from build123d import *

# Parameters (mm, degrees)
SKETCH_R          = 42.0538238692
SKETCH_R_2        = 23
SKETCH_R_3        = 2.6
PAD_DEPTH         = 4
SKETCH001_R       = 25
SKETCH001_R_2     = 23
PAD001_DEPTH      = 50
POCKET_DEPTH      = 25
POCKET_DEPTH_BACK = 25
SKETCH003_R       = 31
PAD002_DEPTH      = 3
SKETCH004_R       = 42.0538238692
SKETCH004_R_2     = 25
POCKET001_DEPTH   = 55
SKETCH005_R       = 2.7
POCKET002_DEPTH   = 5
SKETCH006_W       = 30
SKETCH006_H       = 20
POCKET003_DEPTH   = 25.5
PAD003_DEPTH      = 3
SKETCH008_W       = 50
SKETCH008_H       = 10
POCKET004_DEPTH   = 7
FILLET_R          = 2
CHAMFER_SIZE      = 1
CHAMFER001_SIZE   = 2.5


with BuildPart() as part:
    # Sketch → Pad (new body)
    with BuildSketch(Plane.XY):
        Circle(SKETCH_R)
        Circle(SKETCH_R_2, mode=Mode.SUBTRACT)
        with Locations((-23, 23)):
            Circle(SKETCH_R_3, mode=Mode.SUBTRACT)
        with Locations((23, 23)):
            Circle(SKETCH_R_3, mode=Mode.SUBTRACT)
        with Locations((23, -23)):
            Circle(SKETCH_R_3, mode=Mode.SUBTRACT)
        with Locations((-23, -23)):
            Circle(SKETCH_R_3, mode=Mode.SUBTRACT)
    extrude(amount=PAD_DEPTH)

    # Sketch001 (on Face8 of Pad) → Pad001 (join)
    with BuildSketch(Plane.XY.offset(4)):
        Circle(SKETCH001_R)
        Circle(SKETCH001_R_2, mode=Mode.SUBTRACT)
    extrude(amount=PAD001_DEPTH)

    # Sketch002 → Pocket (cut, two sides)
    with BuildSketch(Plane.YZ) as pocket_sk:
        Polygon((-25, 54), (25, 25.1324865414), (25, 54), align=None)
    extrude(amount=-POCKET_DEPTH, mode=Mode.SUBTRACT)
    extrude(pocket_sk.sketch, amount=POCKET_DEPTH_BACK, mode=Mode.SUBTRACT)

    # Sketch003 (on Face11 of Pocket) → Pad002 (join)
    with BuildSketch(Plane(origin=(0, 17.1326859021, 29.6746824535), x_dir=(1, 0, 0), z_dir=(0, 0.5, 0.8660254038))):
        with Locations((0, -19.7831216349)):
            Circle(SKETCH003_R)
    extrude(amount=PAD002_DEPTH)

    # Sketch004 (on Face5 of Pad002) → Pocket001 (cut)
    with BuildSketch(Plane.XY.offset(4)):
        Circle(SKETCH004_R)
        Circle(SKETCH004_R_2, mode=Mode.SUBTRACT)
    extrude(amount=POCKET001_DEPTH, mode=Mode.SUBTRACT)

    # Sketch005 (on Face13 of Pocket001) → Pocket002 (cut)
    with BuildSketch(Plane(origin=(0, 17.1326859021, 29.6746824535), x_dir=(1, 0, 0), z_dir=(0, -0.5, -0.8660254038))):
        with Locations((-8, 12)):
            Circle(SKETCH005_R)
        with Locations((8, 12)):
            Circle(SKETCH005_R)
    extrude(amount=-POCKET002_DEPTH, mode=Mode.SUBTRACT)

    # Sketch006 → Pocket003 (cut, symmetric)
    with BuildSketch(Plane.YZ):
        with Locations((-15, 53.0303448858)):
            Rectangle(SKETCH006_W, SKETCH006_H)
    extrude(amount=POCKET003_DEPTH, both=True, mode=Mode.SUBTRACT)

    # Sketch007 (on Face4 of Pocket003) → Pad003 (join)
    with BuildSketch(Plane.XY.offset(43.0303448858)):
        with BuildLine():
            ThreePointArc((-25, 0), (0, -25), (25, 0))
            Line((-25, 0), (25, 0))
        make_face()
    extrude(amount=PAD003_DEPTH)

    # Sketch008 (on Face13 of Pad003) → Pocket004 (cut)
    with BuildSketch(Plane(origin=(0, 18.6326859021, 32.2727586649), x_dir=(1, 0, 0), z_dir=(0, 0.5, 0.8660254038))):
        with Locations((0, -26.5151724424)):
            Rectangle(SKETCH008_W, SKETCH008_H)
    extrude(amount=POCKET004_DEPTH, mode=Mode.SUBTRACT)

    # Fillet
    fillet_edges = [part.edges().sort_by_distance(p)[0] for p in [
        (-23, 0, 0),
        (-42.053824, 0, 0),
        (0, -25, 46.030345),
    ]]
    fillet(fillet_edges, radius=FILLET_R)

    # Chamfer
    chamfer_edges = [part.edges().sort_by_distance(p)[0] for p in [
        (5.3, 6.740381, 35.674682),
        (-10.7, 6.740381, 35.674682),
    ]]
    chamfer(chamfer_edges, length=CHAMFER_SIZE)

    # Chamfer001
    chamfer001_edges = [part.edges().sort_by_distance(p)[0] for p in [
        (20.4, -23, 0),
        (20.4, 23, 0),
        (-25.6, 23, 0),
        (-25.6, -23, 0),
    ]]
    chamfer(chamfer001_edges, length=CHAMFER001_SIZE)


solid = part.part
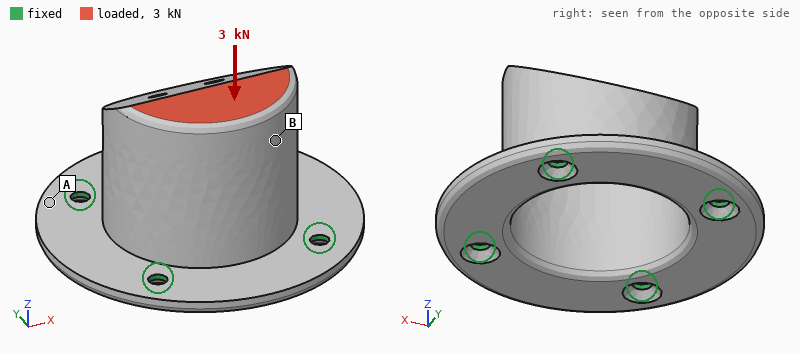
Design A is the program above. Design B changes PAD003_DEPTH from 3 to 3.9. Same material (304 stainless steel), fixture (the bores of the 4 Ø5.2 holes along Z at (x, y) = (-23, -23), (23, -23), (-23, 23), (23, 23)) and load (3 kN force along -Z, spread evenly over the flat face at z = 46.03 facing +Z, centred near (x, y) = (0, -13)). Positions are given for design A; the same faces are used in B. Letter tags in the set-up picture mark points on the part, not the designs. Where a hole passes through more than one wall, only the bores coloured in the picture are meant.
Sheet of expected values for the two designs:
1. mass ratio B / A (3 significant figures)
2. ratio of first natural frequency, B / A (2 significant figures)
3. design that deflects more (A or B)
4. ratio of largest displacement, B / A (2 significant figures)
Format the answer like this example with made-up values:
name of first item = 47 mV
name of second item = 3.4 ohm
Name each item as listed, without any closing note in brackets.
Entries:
mass ratio B / A = 1.02
ratio of first natural frequency, B / A = 0.97
design that deflects more = A
ratio of largest displacement, B / A = 0.90
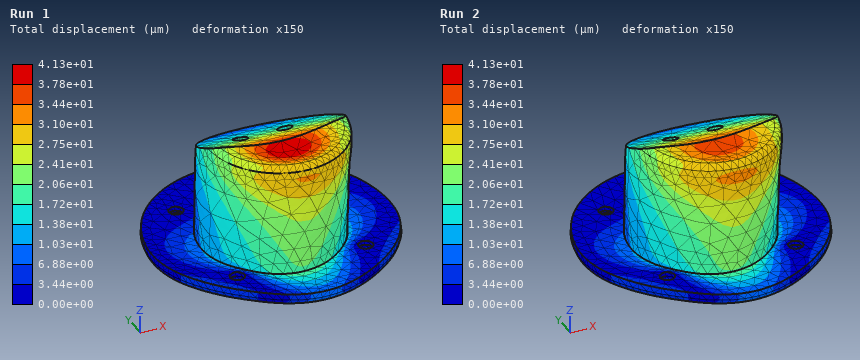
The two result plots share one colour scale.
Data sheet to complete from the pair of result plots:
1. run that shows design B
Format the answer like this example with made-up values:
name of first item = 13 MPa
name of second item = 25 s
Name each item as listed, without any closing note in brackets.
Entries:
run that shows design B = Run 2
